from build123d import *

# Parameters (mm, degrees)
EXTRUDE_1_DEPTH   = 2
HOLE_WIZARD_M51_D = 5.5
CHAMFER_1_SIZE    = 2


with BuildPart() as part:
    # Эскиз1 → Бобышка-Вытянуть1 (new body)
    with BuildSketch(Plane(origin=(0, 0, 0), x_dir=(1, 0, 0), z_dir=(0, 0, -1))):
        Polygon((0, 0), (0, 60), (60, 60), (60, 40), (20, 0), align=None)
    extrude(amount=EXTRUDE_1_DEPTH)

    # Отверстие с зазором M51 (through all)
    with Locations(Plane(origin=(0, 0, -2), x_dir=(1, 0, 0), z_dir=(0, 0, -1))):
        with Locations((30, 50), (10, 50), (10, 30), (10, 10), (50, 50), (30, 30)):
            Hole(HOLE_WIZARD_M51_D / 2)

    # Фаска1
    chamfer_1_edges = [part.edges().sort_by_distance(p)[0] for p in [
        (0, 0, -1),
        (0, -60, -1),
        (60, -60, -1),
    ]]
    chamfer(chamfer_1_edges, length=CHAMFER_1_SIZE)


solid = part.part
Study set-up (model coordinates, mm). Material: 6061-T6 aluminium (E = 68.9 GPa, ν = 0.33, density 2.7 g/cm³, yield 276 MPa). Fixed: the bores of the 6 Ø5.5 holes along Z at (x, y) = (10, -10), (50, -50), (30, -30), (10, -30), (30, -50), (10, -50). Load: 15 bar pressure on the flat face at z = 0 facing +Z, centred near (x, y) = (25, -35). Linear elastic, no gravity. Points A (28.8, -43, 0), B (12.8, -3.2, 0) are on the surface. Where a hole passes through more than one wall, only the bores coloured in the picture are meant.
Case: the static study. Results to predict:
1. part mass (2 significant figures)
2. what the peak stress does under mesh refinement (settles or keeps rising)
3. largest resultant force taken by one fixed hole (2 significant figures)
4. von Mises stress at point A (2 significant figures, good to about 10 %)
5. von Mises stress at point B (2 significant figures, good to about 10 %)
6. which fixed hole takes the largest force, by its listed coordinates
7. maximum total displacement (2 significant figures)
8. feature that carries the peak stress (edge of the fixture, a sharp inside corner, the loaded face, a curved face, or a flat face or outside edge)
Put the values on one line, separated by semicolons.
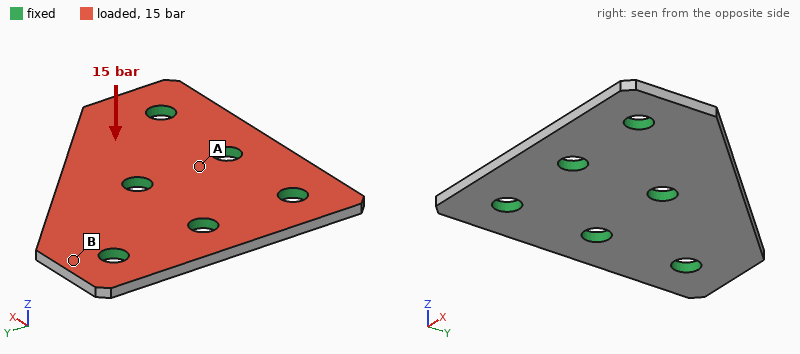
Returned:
14 g; keeps rising; 920 N; 26 MPa; 87 MPa; (30, -30); 0.16 mm; edge of the fixture
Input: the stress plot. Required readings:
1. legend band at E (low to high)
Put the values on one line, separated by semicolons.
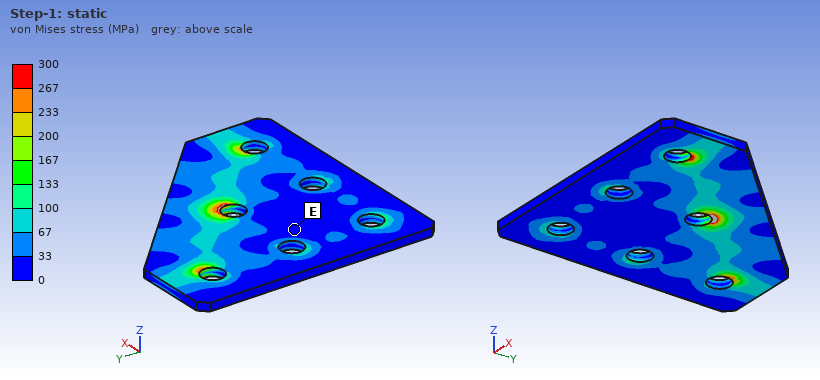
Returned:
0 to 33 MPa
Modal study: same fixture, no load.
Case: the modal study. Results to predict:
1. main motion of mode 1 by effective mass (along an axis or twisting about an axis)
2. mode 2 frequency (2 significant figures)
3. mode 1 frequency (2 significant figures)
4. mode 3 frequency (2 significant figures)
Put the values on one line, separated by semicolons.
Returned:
along Z; 9600 Hz; 8700 Hz; 16 kHz
